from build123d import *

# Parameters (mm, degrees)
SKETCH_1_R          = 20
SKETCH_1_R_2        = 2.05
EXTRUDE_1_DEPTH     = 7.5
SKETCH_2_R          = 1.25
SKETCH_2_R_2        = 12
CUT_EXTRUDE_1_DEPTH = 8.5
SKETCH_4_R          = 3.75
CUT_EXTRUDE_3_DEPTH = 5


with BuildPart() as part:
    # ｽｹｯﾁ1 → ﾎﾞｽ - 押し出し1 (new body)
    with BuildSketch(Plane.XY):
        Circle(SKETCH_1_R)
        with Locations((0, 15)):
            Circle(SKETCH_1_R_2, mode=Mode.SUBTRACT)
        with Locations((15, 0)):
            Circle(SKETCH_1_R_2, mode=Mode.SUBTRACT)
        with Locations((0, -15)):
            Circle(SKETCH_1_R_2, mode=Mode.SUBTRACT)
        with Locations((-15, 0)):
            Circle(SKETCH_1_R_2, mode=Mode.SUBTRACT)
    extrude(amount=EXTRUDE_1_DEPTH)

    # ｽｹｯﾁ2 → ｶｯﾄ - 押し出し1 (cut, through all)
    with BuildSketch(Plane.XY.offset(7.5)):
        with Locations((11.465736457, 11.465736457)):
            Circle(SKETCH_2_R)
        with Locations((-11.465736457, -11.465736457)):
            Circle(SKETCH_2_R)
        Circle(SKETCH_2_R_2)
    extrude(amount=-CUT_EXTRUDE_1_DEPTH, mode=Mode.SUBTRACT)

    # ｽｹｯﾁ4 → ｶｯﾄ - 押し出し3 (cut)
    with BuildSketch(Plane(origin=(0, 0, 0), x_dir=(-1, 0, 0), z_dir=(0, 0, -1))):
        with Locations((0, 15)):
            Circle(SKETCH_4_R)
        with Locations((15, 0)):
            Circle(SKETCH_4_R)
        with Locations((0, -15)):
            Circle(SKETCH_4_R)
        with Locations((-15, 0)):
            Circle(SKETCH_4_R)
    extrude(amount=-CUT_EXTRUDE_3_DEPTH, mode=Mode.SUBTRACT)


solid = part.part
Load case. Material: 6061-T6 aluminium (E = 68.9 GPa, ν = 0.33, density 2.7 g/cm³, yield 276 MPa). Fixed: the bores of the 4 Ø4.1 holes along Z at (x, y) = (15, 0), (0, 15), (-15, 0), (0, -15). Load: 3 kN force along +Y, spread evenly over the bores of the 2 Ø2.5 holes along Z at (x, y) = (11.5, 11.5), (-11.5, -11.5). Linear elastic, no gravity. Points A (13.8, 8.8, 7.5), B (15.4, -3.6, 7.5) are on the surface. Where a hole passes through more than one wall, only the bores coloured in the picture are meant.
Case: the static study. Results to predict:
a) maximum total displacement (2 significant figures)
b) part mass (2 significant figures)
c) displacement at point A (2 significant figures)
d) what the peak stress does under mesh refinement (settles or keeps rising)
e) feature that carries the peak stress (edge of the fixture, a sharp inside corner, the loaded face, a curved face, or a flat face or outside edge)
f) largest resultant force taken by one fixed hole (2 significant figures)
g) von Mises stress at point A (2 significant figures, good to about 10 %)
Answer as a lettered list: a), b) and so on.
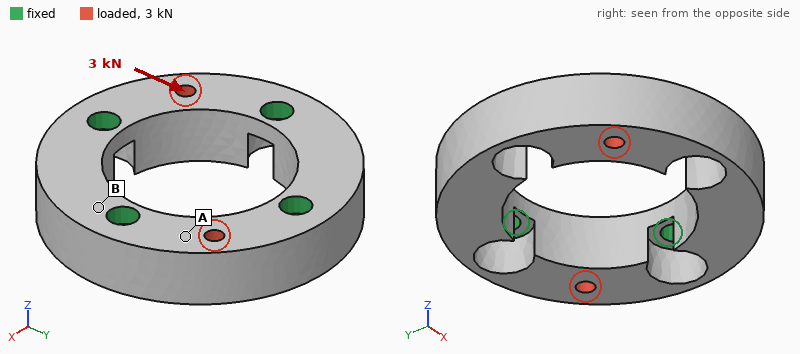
a) 27 µm
b) 13 g
c) 8.3 µm
d) keeps rising
e) a sharp inside corner
f) 1.2 kN
g) 41 MPa
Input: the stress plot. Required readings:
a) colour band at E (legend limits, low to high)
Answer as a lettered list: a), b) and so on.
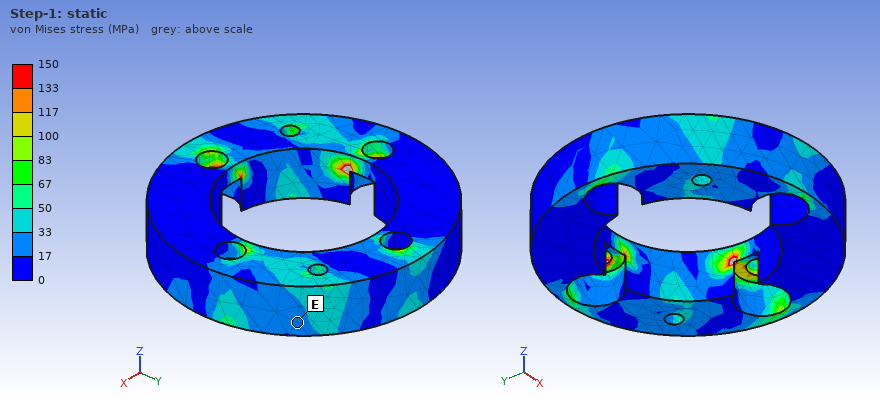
a) 17 to 33 MPa
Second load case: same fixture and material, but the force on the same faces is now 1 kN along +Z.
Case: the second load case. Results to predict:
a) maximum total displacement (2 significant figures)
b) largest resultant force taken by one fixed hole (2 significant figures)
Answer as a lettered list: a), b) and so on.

a) 21 µm
b) 270 N
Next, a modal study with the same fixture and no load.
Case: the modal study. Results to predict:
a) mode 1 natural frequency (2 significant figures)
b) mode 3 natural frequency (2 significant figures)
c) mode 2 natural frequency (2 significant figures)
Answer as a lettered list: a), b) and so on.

a) 16 kHz
b) 19 kHz
c) 19 kHz
